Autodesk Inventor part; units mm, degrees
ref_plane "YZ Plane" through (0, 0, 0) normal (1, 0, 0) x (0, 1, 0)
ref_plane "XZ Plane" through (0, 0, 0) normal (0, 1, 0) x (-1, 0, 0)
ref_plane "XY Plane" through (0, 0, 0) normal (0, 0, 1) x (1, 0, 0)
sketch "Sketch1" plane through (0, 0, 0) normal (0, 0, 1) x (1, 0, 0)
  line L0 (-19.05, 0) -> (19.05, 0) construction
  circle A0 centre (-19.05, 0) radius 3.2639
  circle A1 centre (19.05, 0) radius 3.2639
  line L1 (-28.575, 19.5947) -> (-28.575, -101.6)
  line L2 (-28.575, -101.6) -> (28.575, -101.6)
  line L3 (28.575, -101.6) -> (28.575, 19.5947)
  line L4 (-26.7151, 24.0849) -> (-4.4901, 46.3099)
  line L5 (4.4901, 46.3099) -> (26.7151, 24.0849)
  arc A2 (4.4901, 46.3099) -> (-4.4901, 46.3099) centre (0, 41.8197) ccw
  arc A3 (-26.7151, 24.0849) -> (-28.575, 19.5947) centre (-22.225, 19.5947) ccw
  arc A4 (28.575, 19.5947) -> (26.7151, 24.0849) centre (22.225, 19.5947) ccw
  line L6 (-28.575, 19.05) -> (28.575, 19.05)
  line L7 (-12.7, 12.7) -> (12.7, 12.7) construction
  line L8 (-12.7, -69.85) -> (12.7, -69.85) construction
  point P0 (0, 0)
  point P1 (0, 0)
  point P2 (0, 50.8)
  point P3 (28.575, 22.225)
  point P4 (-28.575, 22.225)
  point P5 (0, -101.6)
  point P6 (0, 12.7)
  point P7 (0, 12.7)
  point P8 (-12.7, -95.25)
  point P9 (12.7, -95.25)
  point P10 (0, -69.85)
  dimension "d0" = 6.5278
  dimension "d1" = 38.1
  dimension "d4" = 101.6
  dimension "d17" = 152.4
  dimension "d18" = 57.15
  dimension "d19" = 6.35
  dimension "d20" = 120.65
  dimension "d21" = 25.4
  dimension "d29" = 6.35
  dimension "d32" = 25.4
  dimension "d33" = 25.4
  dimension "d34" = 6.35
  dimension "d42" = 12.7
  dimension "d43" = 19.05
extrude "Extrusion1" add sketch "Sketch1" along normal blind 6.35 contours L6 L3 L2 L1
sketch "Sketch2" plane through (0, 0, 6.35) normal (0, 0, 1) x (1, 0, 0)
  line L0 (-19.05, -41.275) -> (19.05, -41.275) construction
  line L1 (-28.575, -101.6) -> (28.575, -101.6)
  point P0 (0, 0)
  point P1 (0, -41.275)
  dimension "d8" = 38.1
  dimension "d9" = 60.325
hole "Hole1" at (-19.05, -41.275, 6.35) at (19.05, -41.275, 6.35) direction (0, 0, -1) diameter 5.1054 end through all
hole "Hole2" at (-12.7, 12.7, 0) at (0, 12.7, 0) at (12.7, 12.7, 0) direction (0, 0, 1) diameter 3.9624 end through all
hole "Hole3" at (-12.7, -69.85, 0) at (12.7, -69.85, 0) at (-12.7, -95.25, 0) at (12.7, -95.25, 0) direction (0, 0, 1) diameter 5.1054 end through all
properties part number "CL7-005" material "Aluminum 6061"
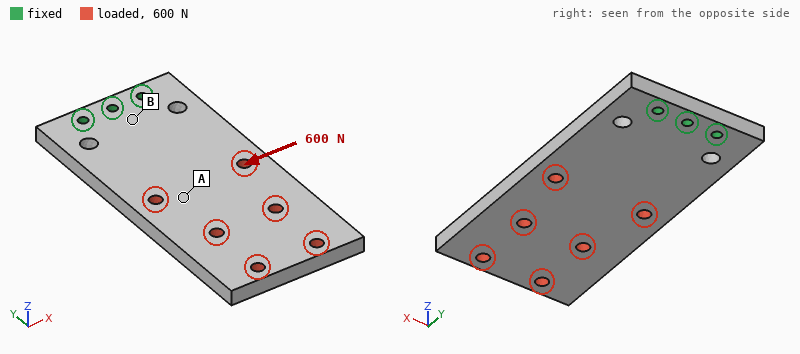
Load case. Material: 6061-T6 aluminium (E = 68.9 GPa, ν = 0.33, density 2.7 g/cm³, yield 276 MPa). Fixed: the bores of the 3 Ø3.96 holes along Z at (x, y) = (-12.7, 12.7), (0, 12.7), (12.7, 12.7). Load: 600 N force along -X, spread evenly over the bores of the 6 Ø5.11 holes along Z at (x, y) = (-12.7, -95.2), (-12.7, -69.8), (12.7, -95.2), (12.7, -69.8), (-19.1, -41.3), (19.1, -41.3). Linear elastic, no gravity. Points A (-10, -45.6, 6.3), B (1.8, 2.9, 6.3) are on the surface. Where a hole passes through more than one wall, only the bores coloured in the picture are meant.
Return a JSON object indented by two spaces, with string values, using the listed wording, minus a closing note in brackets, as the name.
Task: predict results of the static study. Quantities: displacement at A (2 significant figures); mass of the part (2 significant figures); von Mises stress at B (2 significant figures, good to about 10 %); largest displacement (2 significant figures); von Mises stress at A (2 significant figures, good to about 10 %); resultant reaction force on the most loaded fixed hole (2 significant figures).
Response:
{
  "displacement at A": "29 µm",
  "mass of the part": "110 g",
  "von Mises stress at B": "9.9 MPa",
  "largest displacement": "65 µm",
  "von Mises stress at A": "3.9 MPa",
  "resultant reaction force on the most loaded fixed hole": "1.7 kN"
}
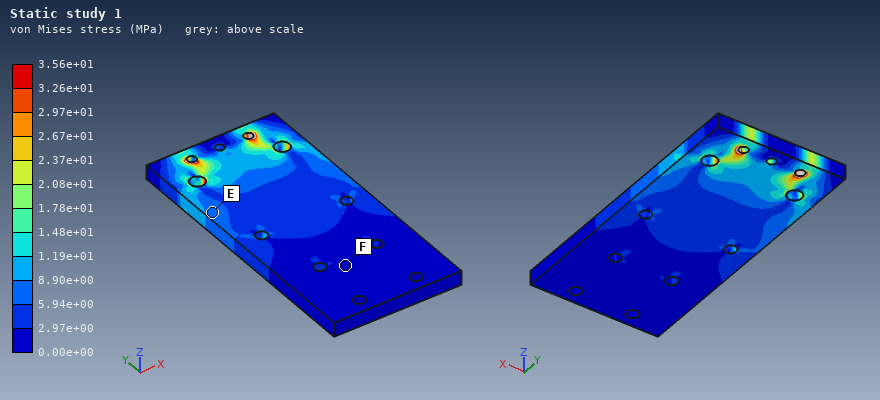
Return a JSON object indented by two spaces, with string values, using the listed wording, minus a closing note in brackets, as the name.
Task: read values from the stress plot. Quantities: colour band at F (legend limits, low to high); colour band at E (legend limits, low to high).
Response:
{
  "colour band at F": "0.00e+00 to 2.97e+00 MPa",
  "colour band at E": "5.94e+00 to 8.90e+00 MPa"
}
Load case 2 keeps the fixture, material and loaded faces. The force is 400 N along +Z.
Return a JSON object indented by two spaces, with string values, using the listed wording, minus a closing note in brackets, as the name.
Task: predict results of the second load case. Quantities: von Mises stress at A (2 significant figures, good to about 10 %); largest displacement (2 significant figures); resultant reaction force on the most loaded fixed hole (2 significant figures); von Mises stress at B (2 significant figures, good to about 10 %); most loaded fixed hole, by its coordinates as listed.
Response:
{
  "von Mises stress at A": "28 MPa",
  "largest displacement": "1.5 mm",
  "resultant reaction force on the most loaded fixed hole": "370 N",
  "von Mises stress at B": "85 MPa",
  "most loaded fixed hole, by its coordinates as listed": "(0, 12.7)"
}
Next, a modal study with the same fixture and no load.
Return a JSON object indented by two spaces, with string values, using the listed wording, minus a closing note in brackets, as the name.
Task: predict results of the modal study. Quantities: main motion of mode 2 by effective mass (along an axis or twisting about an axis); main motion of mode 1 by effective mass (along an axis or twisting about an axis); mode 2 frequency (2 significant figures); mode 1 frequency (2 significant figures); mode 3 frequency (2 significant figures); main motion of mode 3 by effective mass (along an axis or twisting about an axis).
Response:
{
  "main motion of mode 2 by effective mass": "twisting about Y",
  "main motion of mode 1 by effective mass": "along Z",
  "mode 2 frequency": "1600 Hz",
  "mode 1 frequency": "390 Hz",
  "mode 3 frequency": "2200 Hz",
  "main motion of mode 3 by effective mass": "along X"
}
